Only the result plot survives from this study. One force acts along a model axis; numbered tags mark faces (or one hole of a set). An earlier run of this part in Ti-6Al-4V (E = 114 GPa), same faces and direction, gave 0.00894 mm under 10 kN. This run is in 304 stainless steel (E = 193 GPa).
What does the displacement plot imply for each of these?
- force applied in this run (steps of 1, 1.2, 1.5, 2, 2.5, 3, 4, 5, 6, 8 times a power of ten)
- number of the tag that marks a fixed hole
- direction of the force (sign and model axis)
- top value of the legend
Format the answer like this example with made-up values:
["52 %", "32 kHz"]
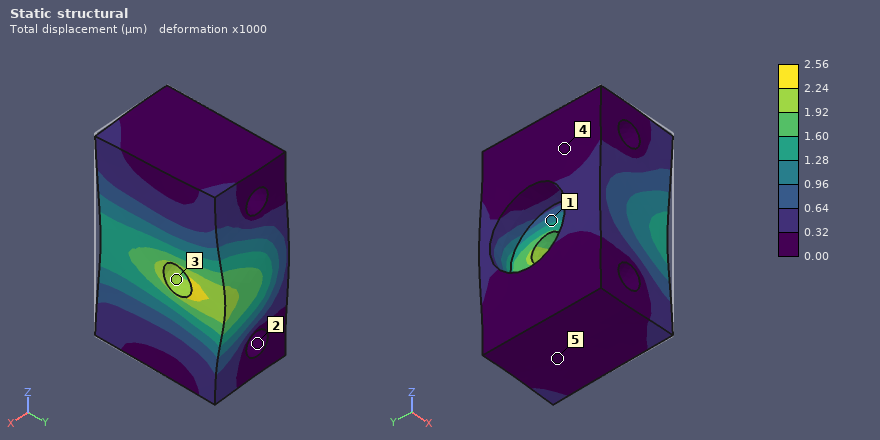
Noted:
["5 kN", "2", "+Y", "2.56 µm"]
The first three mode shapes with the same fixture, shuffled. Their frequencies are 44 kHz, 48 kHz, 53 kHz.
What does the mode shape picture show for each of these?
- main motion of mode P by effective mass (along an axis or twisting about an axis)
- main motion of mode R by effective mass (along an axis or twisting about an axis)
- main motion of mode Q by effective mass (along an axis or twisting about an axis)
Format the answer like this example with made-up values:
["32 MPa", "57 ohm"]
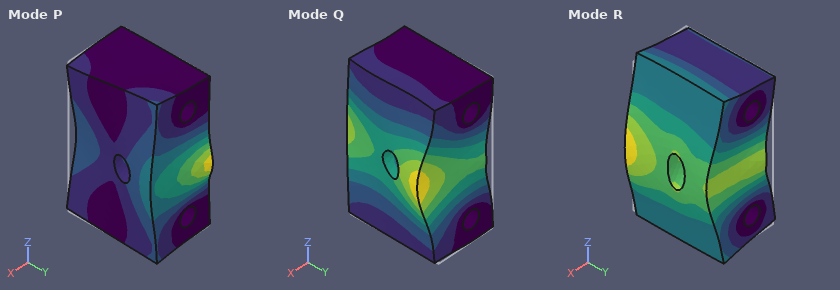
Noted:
["along Y", "along X", "along Y"]
